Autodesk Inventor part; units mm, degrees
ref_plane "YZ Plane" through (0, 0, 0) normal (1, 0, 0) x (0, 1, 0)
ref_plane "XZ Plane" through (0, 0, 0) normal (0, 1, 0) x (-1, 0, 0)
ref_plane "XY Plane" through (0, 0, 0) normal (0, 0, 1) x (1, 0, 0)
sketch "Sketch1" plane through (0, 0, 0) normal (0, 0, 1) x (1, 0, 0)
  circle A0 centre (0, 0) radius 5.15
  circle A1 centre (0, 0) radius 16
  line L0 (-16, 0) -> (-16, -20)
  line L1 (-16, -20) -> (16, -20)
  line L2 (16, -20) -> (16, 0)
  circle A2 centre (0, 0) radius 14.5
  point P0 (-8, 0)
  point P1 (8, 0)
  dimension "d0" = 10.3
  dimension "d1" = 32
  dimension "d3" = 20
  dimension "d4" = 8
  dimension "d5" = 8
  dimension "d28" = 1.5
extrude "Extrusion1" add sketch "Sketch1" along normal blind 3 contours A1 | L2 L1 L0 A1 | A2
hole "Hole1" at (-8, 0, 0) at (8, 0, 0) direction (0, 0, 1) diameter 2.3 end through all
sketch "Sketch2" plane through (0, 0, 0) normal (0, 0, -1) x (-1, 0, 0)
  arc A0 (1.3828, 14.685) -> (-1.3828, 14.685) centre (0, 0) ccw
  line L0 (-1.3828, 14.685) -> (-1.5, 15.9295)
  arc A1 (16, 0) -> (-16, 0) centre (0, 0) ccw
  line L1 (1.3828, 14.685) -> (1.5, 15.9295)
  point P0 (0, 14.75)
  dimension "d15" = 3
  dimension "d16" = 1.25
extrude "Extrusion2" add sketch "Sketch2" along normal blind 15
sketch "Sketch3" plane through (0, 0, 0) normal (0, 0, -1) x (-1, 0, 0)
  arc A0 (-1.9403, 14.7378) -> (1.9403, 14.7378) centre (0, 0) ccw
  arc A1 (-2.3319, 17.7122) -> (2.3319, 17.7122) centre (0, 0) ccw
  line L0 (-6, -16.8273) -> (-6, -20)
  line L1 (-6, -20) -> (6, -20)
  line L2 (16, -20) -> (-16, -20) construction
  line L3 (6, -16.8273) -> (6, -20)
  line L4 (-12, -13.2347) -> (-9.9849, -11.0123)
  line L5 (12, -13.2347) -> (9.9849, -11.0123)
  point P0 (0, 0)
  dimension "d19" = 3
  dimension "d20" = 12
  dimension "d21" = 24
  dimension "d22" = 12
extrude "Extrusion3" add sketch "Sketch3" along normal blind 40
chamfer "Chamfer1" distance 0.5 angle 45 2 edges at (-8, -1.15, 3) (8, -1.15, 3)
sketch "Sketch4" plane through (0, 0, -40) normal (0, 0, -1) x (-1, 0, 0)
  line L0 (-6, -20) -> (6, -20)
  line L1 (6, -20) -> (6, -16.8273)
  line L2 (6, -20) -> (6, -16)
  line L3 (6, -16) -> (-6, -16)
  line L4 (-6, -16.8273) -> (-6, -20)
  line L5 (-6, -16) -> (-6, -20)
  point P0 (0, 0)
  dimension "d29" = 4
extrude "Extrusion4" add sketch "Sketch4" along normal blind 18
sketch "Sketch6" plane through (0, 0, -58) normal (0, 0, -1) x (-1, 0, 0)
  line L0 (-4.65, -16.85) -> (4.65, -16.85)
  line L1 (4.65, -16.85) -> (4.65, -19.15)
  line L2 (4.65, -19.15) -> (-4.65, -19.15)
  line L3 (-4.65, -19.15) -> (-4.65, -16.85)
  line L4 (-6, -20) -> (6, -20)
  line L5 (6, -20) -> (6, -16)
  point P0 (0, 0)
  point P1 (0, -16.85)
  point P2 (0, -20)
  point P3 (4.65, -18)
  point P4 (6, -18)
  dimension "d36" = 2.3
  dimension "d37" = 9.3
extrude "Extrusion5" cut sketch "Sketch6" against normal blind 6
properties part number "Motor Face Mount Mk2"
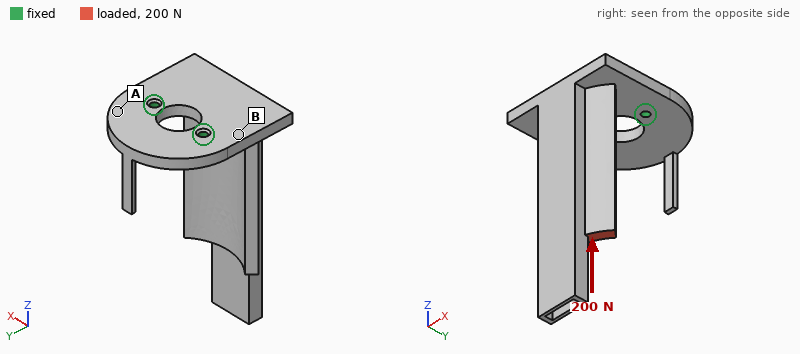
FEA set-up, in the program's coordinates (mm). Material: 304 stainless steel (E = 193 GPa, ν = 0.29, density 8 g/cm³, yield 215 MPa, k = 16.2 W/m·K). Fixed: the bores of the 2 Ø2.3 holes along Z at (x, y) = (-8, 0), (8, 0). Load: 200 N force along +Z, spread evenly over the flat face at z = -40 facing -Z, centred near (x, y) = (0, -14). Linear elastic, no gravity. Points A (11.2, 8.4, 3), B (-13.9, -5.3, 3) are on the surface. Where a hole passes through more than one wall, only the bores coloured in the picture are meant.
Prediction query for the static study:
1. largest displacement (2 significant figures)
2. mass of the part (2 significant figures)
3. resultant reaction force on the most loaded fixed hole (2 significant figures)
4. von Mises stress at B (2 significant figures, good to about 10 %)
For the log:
0.13 mm
62 g
100 N
42 MPa
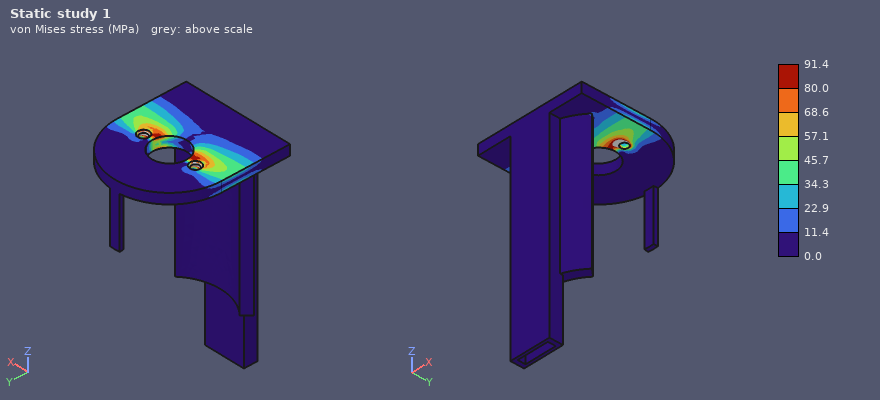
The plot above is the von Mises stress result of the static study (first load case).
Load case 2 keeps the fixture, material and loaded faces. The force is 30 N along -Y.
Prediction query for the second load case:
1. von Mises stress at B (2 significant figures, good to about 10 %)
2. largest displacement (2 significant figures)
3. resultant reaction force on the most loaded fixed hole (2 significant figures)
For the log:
29 MPa
0.12 mm
16 N
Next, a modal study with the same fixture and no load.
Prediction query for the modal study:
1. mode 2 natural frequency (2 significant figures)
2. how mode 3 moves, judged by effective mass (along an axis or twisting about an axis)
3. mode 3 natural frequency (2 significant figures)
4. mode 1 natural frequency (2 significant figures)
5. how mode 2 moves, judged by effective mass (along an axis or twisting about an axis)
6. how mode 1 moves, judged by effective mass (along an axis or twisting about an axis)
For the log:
1500 Hz
along Z
3700 Hz
660 Hz
along X
along Y
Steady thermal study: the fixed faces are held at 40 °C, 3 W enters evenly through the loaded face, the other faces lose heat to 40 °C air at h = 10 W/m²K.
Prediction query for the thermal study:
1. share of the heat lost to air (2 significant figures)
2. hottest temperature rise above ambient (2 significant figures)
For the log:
53 %
76 K
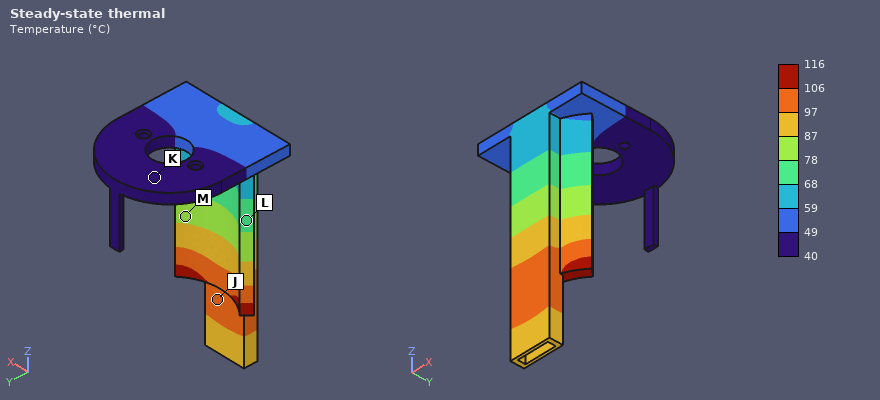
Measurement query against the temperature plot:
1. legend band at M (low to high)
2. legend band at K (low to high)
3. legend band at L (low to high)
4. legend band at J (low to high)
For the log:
78 to 87 °C
40 to 49 °C
68 to 78 °C
97 to 106 °C
